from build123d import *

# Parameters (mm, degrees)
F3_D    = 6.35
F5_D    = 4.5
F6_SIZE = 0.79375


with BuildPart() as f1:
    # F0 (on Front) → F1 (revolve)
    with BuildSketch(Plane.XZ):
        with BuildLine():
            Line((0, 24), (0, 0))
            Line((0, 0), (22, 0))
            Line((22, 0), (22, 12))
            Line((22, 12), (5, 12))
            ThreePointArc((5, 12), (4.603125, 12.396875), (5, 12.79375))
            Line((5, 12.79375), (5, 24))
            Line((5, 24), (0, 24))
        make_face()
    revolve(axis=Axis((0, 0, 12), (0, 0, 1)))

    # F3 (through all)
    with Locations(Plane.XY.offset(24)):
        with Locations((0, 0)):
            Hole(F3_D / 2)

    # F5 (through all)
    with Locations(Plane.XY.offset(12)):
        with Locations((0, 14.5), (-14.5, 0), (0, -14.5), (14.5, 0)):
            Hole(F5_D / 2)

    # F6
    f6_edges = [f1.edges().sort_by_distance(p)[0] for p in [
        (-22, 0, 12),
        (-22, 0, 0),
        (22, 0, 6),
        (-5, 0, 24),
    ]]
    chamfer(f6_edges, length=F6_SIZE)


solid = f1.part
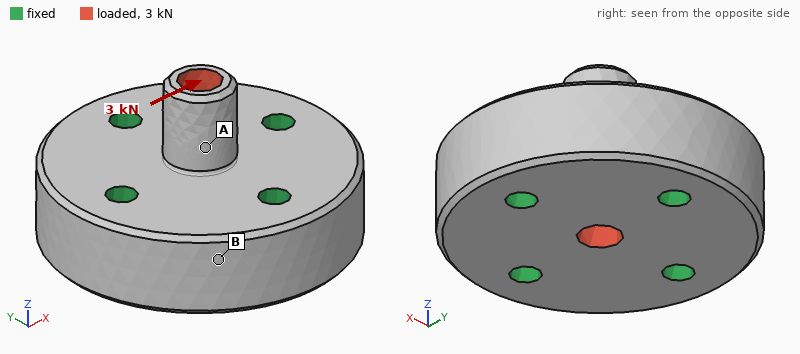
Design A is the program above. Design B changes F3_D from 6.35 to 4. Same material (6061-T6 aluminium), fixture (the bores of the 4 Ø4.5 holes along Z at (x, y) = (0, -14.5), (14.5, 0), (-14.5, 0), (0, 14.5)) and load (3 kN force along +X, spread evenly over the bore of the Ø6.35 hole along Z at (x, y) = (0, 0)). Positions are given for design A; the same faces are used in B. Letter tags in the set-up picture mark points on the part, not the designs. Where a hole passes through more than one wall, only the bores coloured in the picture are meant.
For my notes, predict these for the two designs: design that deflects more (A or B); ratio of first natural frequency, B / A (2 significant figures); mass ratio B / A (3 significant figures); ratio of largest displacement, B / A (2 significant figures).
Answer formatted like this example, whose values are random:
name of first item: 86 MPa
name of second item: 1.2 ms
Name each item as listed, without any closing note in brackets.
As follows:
design that deflects more: A
ratio of first natural frequency, B / A: 0.97
mass ratio B / A: 1.03
ratio of largest displacement, B / A: 0.76
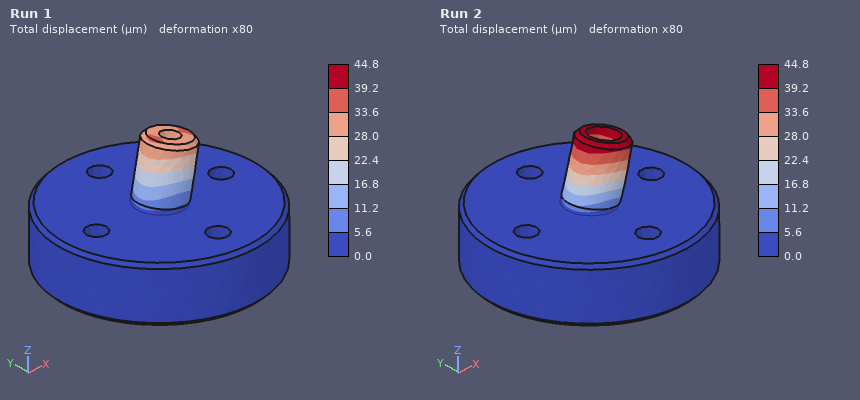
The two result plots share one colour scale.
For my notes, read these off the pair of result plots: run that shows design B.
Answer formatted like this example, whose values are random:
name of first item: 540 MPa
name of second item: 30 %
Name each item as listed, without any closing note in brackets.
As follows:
run that shows design B: Run 1
